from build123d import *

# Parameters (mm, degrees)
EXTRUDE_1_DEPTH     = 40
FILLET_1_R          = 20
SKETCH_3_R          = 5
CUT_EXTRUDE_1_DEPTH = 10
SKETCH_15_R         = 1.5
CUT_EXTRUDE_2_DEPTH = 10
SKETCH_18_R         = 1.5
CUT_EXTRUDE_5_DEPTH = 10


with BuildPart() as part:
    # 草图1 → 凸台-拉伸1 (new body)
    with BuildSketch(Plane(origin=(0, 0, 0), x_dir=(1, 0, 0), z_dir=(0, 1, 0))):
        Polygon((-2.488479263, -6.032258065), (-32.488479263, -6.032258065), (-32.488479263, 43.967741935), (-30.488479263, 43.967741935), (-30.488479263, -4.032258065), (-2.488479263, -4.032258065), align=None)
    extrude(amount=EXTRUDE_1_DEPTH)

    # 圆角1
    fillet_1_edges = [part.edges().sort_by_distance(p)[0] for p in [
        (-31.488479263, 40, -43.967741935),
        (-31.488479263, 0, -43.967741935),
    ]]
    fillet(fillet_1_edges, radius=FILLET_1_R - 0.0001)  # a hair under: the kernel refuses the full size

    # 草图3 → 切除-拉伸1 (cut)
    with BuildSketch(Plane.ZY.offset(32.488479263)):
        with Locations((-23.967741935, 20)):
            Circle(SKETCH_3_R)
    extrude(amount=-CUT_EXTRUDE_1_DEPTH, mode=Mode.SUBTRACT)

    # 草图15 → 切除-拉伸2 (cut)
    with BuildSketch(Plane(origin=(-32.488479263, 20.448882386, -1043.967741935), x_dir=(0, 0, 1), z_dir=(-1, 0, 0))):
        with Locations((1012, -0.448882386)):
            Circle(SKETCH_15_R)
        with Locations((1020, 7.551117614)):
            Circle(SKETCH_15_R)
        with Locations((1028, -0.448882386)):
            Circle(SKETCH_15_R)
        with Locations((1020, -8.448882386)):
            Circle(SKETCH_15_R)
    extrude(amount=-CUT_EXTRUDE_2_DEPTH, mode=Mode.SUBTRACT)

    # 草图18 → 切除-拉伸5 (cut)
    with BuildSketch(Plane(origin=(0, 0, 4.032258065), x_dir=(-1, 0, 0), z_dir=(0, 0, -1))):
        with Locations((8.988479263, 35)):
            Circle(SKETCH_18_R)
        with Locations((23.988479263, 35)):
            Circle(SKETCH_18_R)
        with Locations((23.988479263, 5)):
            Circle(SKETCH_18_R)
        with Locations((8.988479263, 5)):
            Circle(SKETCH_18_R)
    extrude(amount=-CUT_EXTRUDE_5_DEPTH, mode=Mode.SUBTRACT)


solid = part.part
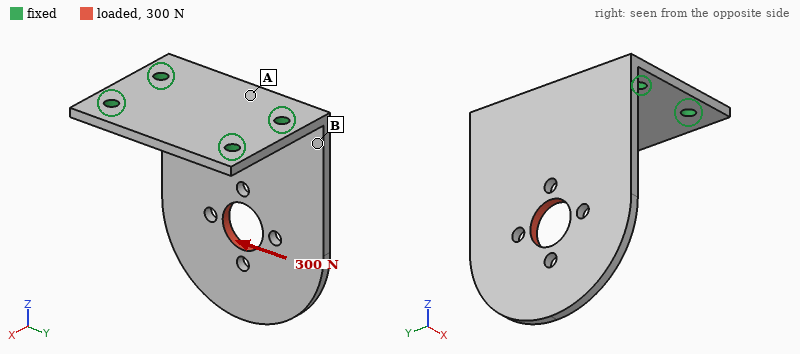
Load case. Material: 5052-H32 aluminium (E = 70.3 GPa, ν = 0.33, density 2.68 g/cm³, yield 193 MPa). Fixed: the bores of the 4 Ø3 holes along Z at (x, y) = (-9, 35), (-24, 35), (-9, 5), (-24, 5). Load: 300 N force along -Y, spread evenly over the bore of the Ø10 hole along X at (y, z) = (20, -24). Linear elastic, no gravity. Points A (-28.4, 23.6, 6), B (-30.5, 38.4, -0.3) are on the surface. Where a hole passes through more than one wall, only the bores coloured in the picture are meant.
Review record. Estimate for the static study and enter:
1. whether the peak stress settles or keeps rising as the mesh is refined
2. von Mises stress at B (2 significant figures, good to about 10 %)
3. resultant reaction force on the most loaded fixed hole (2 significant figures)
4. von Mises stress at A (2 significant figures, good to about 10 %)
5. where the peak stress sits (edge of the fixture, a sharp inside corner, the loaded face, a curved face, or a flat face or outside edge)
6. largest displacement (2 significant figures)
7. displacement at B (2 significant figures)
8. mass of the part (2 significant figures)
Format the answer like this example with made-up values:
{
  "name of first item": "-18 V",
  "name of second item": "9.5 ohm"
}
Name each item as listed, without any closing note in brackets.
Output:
{
  "whether the peak stress settles or keeps rising as the mesh is refined": "keeps rising",
  "von Mises stress at B": "51 MPa",
  "resultant reaction force on the most loaded fixed hole": "330 N",
  "von Mises stress at A": "24 MPa",
  "where the peak stress sits": "edge of the fixture",
  "largest displacement": "0.14 mm",
  "displacement at B": "0.056 mm",
  "mass of the part": "15 g"
}
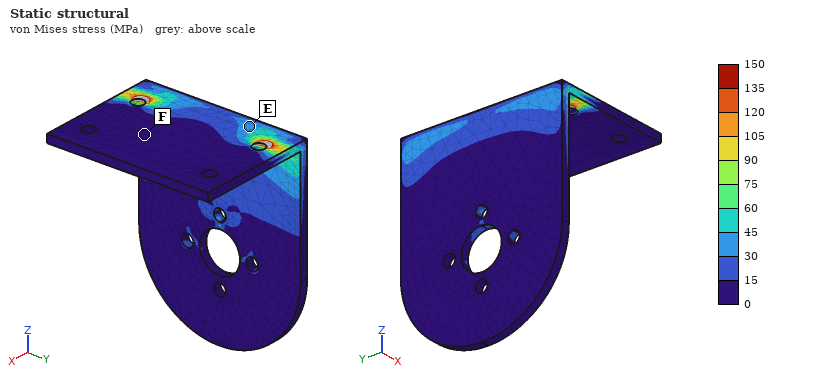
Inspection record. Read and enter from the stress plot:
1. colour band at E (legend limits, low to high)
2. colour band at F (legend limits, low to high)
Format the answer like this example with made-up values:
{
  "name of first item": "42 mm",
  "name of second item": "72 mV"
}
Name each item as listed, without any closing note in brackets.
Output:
{
  "colour band at E": "30 to 45 MPa",
  "colour band at F": "0 to 15 MPa"
}
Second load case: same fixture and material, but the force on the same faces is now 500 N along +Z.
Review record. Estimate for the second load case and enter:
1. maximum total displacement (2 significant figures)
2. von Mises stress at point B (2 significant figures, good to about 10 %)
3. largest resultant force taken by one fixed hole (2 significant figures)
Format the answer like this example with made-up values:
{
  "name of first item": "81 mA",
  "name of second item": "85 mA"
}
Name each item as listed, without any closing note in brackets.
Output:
{
  "maximum total displacement": "0.37 mm",
  "von Mises stress at point B": "19 MPa",
  "largest resultant force taken by one fixed hole": "280 N"
}
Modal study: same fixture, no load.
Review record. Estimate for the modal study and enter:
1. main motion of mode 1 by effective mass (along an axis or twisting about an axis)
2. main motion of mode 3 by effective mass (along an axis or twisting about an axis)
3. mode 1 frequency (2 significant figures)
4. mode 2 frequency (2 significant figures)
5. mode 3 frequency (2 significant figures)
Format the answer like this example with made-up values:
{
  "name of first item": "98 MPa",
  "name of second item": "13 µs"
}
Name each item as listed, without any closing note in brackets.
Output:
{
  "main motion of mode 1 by effective mass": "along X",
  "main motion of mode 3 by effective mass": "along Y",
  "mode 1 frequency": "670 Hz",
  "mode 2 frequency": "2100 Hz",
  "mode 3 frequency": "3600 Hz"
}
